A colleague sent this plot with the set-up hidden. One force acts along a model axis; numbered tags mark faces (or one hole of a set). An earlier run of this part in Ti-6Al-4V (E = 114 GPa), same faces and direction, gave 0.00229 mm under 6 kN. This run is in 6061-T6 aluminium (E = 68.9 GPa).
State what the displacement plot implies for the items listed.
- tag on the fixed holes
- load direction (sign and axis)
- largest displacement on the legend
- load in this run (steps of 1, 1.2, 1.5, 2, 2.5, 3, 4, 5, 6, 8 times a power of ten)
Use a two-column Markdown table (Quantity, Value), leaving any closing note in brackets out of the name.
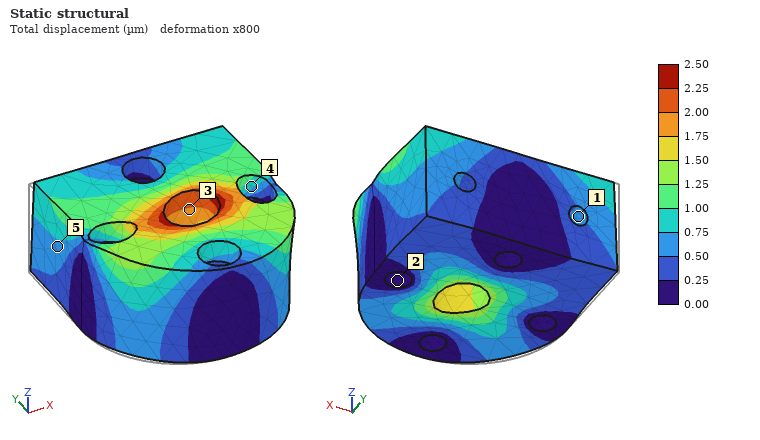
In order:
| Quantity | Value |
|---|---|
| tag on the fixed holes | 2 |
| load direction | +X |
| largest displacement on the legend | 2.50 µm |
| load in this run | 4 kN |
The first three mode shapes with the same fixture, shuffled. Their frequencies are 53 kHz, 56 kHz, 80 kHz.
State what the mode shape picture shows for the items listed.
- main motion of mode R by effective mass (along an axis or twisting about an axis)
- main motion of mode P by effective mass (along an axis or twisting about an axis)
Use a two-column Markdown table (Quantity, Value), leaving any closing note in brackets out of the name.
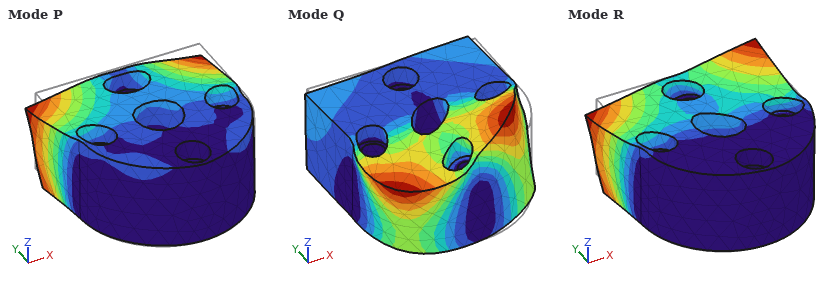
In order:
| Quantity | Value |
|---|---|
| main motion of mode R by effective mass | twisting about Y |
| main motion of mode P by effective mass | along Z |
